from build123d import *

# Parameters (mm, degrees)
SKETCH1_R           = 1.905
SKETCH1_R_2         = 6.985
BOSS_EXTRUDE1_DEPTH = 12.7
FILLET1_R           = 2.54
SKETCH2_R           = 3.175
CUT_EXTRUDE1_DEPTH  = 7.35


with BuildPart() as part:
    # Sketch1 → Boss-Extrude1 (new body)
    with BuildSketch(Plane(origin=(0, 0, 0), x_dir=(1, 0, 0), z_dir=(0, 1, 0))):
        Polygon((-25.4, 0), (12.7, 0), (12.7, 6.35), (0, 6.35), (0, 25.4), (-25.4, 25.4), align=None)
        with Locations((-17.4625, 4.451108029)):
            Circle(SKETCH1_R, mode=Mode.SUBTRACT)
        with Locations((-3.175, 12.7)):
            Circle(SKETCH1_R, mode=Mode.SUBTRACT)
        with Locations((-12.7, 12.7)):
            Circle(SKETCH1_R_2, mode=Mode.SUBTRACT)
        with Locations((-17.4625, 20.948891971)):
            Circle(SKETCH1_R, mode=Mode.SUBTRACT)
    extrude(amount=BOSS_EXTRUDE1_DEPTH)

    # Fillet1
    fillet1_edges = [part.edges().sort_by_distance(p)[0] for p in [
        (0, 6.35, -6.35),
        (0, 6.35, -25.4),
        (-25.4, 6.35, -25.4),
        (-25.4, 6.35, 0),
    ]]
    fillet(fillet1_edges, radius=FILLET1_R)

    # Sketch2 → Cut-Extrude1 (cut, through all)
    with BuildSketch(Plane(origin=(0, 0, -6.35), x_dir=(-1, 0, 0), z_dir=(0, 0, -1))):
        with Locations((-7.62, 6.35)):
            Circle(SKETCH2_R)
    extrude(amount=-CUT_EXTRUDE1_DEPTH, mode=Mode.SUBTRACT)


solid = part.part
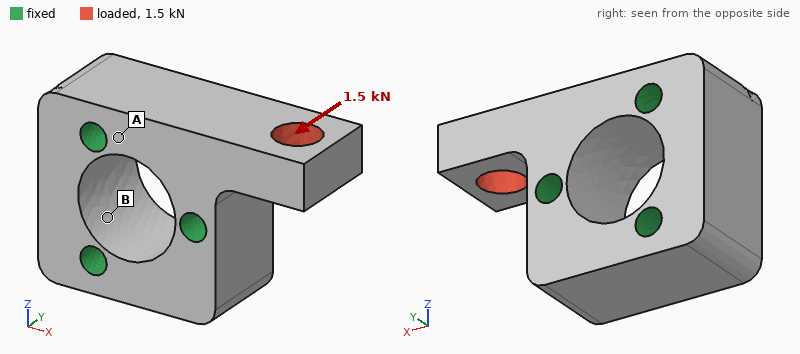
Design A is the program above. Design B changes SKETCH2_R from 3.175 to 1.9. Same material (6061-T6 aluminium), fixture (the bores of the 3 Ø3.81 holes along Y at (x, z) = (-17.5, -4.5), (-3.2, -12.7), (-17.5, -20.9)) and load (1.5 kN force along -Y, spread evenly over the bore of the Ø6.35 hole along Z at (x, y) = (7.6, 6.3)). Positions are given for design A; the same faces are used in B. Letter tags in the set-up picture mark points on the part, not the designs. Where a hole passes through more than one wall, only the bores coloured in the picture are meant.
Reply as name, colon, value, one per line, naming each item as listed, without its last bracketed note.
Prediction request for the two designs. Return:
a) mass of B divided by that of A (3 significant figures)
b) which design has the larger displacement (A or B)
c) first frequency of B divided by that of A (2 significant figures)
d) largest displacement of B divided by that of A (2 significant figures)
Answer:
mass of B divided by that of A: 1.02
which design has the larger displacement: A
first frequency of B divided by that of A: 0.99
largest displacement of B divided by that of A: 0.83
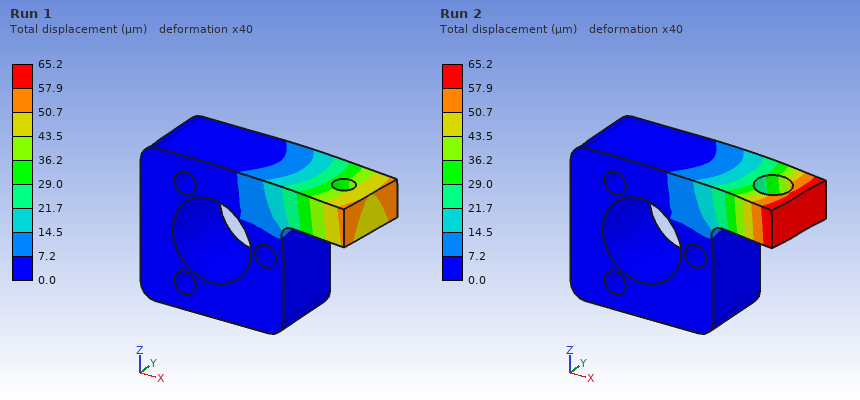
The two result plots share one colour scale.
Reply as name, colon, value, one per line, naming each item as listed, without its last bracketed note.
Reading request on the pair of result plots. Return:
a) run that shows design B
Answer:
run that shows design B: Run 1
